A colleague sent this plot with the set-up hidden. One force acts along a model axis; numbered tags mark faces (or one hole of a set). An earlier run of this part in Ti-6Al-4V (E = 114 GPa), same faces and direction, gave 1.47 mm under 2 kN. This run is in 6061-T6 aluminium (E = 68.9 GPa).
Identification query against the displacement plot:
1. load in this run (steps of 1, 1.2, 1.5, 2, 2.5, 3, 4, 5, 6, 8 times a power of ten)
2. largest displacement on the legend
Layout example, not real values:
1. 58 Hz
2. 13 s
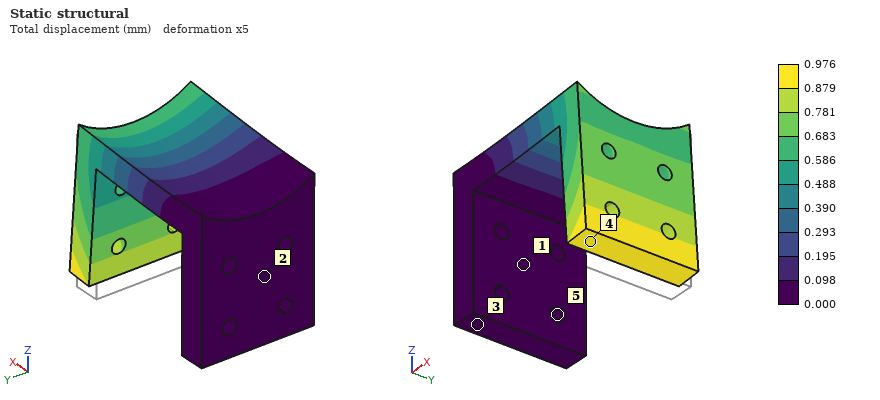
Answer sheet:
1. 800 N
2. 0.976 mm
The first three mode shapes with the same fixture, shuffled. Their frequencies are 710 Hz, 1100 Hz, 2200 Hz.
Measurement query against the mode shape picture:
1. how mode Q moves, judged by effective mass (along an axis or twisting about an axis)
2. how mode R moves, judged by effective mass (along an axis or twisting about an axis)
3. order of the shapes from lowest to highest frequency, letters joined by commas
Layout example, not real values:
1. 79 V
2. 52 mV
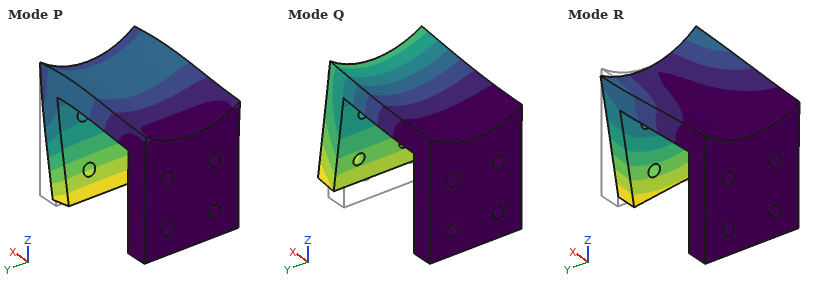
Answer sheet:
1. along Z
2. along Y
3. Q, R, P
